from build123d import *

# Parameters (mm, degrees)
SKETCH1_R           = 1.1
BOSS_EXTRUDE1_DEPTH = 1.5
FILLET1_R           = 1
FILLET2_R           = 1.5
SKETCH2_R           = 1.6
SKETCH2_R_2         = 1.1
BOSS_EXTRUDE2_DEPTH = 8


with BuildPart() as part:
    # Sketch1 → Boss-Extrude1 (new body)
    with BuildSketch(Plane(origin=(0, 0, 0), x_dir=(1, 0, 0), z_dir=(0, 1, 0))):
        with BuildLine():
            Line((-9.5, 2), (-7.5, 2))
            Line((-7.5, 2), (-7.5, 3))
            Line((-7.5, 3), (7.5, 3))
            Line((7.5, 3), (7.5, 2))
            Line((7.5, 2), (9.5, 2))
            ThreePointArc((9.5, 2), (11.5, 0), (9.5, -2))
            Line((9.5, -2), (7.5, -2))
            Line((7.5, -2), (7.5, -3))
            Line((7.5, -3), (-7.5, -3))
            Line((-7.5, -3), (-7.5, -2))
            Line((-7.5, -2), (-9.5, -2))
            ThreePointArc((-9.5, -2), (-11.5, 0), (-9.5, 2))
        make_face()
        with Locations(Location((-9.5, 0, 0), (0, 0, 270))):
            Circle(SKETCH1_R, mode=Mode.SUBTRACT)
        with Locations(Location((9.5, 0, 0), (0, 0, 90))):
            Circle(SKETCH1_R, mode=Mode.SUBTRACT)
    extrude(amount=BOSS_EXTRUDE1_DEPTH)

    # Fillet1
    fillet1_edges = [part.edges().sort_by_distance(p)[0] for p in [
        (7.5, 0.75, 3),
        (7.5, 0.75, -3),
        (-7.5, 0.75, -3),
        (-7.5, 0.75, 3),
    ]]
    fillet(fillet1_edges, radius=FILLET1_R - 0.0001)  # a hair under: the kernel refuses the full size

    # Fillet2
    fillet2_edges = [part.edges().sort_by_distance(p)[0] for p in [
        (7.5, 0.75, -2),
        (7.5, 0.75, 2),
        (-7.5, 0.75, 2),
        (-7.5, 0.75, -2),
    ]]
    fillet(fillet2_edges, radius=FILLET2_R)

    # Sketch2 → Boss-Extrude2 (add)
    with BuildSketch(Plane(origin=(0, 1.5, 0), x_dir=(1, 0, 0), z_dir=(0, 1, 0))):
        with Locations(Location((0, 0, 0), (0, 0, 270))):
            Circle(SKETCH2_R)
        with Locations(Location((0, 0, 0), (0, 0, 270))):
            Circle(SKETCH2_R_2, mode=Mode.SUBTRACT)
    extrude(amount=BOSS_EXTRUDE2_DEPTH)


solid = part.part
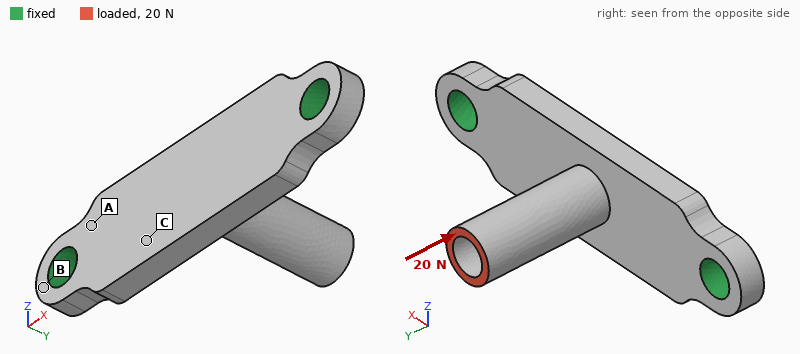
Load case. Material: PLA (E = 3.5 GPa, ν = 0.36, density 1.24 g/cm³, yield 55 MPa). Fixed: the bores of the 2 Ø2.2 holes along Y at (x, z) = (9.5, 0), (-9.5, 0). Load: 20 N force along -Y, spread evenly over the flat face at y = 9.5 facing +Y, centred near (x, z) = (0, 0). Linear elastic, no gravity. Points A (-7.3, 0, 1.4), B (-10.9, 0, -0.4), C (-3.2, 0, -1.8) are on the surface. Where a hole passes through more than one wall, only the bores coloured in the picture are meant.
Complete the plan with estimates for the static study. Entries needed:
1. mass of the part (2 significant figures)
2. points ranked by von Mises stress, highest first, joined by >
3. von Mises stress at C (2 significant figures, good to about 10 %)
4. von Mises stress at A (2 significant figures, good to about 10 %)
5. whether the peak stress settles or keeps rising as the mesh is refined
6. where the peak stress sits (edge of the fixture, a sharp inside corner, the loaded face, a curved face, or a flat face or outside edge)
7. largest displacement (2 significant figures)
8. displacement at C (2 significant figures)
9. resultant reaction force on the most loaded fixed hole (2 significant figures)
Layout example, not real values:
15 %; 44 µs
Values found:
0.25 g; A > C > B; 7.0 MPa; 13 MPa; keeps rising; edge of the fixture; 0.11 mm; 0.076 mm; 10 N
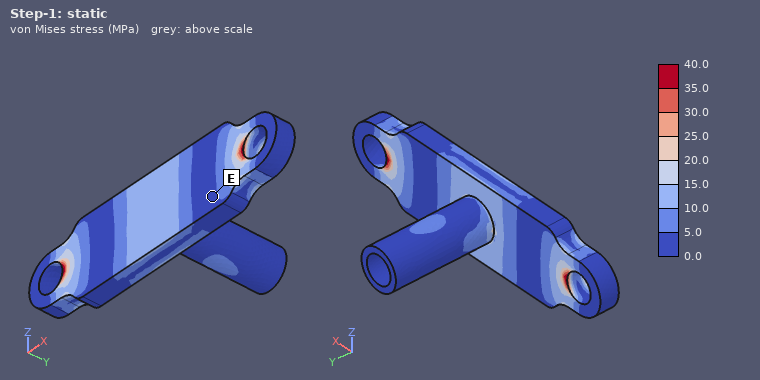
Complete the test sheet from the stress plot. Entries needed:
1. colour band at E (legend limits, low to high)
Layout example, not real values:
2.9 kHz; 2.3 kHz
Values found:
0.0 to 5.0 MPa
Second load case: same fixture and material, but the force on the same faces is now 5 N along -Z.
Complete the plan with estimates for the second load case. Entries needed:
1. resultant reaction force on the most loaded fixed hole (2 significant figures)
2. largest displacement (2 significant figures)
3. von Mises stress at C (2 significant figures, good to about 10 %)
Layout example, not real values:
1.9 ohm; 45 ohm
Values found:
2.5 N; 0.29 mm; 7.0 MPa
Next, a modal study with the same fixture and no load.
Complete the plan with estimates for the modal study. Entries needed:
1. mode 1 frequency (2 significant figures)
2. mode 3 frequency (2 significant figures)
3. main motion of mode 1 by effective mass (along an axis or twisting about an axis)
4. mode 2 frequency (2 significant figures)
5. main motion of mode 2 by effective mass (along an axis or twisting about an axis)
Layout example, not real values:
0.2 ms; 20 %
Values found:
5100 Hz; 8100 Hz; along Z; 6300 Hz; along Y
